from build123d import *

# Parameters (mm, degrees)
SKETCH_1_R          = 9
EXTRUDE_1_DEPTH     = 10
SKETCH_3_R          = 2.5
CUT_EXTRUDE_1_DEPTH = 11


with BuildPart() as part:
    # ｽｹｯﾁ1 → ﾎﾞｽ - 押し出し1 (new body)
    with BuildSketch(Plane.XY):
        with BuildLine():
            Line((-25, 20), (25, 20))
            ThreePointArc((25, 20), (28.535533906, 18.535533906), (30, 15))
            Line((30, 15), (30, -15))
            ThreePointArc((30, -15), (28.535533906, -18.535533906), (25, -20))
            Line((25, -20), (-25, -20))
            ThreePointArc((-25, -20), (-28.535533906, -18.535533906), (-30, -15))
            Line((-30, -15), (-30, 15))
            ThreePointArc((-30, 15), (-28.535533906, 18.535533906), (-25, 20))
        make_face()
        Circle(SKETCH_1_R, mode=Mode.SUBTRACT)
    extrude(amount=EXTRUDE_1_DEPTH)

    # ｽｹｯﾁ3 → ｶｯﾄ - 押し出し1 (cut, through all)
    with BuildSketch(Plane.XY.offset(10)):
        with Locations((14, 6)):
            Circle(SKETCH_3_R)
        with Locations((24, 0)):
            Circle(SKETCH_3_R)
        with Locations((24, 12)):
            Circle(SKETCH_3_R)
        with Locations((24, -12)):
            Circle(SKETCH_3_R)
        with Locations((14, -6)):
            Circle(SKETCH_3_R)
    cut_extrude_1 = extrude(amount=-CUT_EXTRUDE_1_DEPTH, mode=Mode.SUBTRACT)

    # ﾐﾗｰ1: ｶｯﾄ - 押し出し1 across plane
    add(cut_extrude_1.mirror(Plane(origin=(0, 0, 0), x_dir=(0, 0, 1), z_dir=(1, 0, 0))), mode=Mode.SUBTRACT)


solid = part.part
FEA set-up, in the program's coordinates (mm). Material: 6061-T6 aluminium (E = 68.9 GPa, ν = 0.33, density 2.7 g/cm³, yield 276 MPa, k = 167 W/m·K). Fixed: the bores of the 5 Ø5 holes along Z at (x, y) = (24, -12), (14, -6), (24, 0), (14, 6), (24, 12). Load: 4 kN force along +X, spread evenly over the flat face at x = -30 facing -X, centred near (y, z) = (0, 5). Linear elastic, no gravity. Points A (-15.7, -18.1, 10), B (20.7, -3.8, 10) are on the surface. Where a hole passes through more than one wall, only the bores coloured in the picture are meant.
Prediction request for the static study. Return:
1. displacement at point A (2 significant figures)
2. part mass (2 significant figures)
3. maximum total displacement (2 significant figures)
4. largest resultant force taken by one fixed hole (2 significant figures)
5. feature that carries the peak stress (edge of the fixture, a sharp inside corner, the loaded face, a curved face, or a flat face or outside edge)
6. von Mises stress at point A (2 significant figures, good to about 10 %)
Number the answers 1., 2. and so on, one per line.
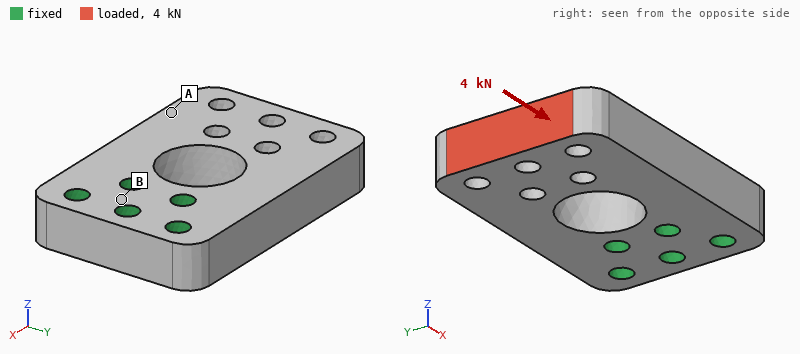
1. 7.8 µm
2. 52 g
3. 16 µm
4. 1.2 kN
5. a curved face
6. 9.6 MPa
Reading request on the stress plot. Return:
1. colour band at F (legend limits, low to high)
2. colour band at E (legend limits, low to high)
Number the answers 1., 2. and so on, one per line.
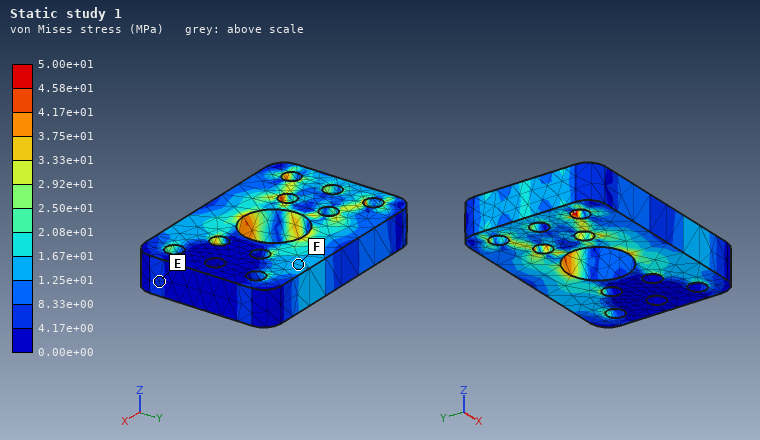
1. 1.25e+01 to 1.67e+01 MPa
2. 4.17e+00 to 8.33e+00 MPa
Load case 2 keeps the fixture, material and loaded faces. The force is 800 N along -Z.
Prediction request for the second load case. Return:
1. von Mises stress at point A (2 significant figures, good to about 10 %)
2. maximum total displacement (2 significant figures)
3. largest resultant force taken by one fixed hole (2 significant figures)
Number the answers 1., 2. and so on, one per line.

1. 24 MPa
2. 0.18 mm
3. 880 N
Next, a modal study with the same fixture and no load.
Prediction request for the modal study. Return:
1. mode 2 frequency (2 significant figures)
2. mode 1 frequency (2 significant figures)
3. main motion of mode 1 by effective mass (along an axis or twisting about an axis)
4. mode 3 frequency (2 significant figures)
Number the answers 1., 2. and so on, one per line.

1. 7700 Hz
2. 3400 Hz
3. along Z
4. 7800 Hz
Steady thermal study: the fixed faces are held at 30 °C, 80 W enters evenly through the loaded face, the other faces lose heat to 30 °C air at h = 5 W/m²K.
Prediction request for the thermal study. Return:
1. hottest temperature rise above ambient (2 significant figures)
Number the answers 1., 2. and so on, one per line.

1. 85 K
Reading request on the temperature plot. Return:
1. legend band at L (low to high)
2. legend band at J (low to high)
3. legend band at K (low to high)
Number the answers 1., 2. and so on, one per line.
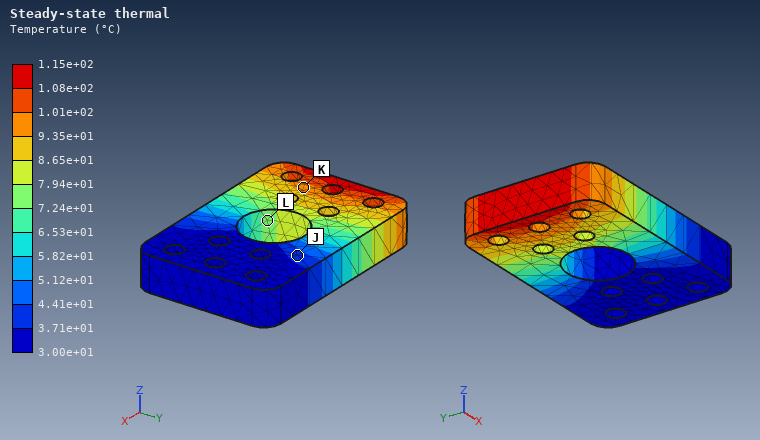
1. 7.24e+01 to 7.94e+01 °C
2. 3.71e+01 to 4.41e+01 °C
3. 9.35e+01 to 1.01e+02 °C
